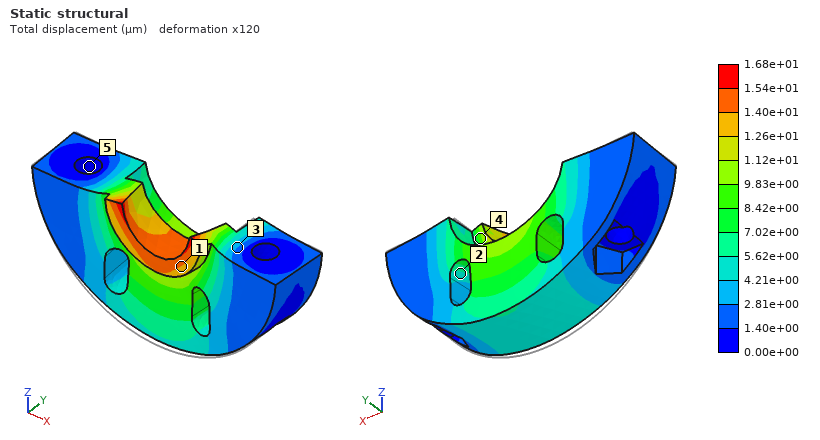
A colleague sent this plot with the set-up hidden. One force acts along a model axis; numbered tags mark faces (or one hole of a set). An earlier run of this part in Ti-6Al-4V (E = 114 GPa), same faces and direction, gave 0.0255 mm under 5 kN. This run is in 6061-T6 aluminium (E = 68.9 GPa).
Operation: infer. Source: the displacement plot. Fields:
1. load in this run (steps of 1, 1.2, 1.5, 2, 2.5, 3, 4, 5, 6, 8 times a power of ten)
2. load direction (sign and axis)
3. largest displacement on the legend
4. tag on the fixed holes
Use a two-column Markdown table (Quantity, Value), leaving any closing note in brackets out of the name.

| Quantity | Value |
|---|---|
| load in this run | 2 kN |
| load direction | +Y |
| largest displacement on the legend | 1.68e+01 µm |
| tag on the fixed holes | 5 |
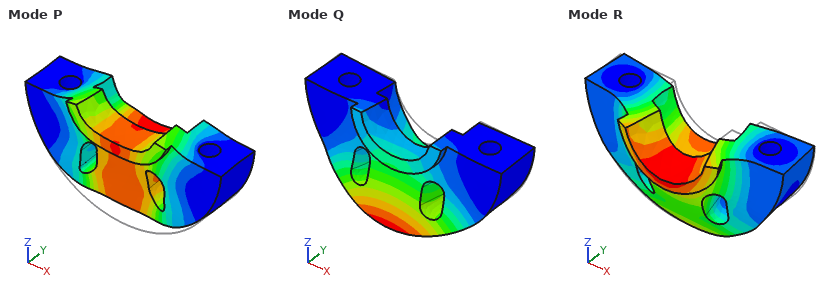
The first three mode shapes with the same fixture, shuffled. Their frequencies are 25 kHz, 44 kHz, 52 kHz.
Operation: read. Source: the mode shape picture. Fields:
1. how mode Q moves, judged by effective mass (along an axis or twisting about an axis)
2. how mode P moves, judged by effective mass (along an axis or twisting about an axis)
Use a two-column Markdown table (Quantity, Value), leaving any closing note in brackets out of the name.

| Quantity | Value |
|---|---|
| how mode Q moves, judged by effective mass | along Y |
| how mode P moves, judged by effective mass | along Z |
